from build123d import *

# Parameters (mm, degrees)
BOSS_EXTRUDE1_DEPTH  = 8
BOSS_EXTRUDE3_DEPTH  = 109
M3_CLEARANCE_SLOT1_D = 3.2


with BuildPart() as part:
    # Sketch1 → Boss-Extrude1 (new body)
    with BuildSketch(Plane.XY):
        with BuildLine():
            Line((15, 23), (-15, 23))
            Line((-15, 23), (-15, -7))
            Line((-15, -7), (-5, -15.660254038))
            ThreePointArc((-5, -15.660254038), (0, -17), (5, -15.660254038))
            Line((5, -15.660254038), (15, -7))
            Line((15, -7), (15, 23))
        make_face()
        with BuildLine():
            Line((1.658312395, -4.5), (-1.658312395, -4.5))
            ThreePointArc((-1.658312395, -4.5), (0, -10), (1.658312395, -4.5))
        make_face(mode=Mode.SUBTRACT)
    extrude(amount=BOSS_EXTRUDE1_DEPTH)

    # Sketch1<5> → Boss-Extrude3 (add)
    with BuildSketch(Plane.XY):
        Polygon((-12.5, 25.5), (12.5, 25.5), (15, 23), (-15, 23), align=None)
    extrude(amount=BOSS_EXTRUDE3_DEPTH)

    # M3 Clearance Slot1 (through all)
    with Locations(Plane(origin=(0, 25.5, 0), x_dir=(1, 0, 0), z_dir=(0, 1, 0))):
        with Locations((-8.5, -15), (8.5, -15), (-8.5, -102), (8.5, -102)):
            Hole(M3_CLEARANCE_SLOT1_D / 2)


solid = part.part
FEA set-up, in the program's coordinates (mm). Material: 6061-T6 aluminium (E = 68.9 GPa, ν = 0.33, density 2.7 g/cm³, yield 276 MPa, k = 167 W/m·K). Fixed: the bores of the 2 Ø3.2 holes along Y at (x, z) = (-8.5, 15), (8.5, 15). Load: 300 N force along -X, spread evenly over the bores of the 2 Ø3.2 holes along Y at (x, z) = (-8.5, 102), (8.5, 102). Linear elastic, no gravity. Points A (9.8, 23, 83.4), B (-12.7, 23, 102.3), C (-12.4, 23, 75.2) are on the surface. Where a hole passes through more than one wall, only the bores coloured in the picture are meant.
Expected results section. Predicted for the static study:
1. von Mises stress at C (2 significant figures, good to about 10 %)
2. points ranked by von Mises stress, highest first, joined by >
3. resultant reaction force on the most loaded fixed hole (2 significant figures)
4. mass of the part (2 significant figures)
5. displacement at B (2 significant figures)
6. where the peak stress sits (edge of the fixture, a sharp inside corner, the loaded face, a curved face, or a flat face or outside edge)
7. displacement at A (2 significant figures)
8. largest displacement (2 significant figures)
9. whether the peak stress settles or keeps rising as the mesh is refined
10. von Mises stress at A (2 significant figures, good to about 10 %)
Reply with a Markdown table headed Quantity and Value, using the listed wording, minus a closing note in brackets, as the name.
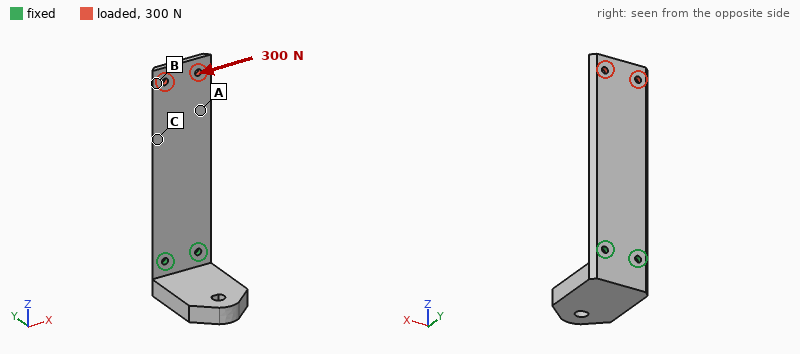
| Quantity | Value |
|---|---|
| von Mises stress at C | 23 MPa |
| points ranked by von Mises stress, highest first, joined by > | C > A > B |
| resultant reaction force on the most loaded fixed hole | 1.4 kN |
| mass of the part | 43 g |
| displacement at B | 0.25 mm |
| where the peak stress sits | edge of the fixture |
| displacement at A | 0.18 mm |
| largest displacement | 0.28 mm |
| whether the peak stress settles or keeps rising as the mesh is refined | keeps rising |
| von Mises stress at A | 14 MPa |
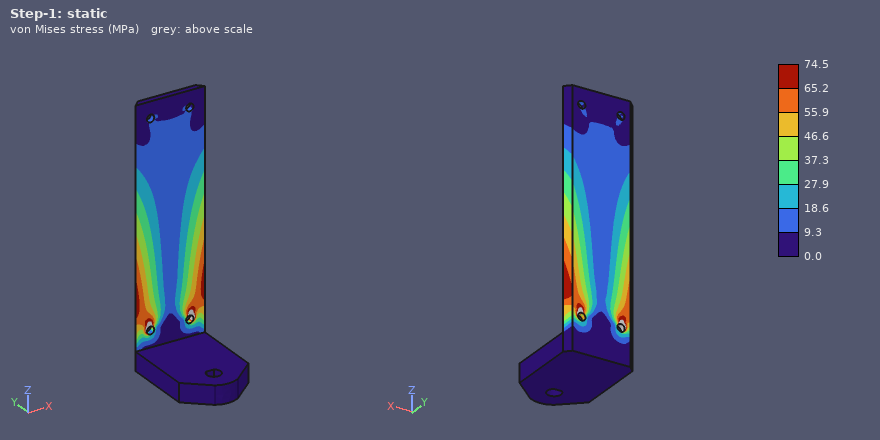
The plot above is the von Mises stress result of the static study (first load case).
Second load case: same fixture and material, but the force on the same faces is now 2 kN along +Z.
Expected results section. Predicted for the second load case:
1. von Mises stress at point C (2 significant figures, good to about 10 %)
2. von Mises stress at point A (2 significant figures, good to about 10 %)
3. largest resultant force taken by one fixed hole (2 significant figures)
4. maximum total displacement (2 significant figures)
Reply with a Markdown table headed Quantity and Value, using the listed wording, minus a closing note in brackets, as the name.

| Quantity | Value |
|---|---|
| von Mises stress at point C | 27 MPa |
| von Mises stress at point A | 27 MPa |
| largest resultant force taken by one fixed hole | 1.0 kN |
| maximum total displacement | 0.13 mm |
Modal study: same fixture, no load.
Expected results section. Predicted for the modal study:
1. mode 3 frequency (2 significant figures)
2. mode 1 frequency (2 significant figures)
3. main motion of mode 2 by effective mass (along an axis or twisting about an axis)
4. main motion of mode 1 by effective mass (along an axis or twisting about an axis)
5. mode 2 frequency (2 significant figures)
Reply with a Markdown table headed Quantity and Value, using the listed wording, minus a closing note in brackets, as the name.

| Quantity | Value |
|---|---|
| mode 3 frequency | 1500 Hz |
| mode 1 frequency | 240 Hz |
| main motion of mode 2 by effective mass | along Z |
| main motion of mode 1 by effective mass | along Y |
| mode 2 frequency | 820 Hz |
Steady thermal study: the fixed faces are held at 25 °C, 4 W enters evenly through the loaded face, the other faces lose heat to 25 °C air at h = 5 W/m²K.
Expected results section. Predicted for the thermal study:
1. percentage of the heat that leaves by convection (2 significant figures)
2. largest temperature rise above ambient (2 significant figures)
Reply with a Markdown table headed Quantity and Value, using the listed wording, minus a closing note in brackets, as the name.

| Quantity | Value |
|---|---|
| percentage of the heat that leaves by convection | 11 % |
| largest temperature rise above ambient | 29 K |
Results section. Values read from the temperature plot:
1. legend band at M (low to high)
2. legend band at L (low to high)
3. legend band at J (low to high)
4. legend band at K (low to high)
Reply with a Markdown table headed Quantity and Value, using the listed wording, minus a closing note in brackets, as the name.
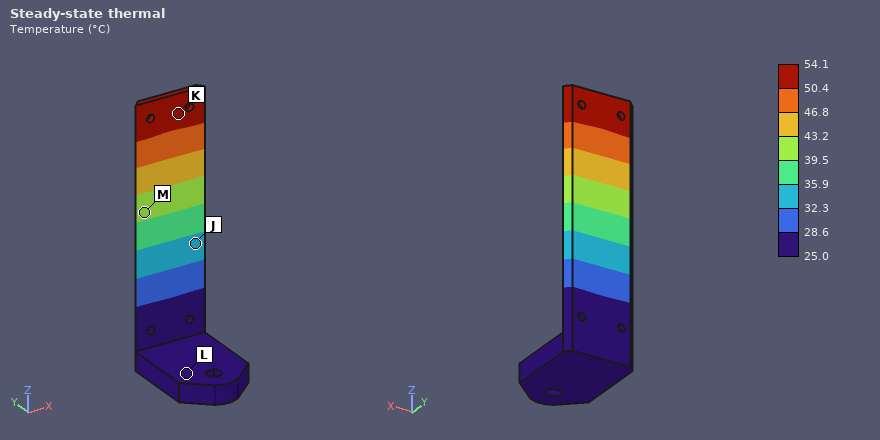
| Quantity | Value |
|---|---|
| legend band at M | 39.5 to 43.2 °C |
| legend band at L | 25.0 to 28.6 °C |
| legend band at J | 32.3 to 35.9 °C |
| legend band at K | 50.4 to 54.1 °C |
